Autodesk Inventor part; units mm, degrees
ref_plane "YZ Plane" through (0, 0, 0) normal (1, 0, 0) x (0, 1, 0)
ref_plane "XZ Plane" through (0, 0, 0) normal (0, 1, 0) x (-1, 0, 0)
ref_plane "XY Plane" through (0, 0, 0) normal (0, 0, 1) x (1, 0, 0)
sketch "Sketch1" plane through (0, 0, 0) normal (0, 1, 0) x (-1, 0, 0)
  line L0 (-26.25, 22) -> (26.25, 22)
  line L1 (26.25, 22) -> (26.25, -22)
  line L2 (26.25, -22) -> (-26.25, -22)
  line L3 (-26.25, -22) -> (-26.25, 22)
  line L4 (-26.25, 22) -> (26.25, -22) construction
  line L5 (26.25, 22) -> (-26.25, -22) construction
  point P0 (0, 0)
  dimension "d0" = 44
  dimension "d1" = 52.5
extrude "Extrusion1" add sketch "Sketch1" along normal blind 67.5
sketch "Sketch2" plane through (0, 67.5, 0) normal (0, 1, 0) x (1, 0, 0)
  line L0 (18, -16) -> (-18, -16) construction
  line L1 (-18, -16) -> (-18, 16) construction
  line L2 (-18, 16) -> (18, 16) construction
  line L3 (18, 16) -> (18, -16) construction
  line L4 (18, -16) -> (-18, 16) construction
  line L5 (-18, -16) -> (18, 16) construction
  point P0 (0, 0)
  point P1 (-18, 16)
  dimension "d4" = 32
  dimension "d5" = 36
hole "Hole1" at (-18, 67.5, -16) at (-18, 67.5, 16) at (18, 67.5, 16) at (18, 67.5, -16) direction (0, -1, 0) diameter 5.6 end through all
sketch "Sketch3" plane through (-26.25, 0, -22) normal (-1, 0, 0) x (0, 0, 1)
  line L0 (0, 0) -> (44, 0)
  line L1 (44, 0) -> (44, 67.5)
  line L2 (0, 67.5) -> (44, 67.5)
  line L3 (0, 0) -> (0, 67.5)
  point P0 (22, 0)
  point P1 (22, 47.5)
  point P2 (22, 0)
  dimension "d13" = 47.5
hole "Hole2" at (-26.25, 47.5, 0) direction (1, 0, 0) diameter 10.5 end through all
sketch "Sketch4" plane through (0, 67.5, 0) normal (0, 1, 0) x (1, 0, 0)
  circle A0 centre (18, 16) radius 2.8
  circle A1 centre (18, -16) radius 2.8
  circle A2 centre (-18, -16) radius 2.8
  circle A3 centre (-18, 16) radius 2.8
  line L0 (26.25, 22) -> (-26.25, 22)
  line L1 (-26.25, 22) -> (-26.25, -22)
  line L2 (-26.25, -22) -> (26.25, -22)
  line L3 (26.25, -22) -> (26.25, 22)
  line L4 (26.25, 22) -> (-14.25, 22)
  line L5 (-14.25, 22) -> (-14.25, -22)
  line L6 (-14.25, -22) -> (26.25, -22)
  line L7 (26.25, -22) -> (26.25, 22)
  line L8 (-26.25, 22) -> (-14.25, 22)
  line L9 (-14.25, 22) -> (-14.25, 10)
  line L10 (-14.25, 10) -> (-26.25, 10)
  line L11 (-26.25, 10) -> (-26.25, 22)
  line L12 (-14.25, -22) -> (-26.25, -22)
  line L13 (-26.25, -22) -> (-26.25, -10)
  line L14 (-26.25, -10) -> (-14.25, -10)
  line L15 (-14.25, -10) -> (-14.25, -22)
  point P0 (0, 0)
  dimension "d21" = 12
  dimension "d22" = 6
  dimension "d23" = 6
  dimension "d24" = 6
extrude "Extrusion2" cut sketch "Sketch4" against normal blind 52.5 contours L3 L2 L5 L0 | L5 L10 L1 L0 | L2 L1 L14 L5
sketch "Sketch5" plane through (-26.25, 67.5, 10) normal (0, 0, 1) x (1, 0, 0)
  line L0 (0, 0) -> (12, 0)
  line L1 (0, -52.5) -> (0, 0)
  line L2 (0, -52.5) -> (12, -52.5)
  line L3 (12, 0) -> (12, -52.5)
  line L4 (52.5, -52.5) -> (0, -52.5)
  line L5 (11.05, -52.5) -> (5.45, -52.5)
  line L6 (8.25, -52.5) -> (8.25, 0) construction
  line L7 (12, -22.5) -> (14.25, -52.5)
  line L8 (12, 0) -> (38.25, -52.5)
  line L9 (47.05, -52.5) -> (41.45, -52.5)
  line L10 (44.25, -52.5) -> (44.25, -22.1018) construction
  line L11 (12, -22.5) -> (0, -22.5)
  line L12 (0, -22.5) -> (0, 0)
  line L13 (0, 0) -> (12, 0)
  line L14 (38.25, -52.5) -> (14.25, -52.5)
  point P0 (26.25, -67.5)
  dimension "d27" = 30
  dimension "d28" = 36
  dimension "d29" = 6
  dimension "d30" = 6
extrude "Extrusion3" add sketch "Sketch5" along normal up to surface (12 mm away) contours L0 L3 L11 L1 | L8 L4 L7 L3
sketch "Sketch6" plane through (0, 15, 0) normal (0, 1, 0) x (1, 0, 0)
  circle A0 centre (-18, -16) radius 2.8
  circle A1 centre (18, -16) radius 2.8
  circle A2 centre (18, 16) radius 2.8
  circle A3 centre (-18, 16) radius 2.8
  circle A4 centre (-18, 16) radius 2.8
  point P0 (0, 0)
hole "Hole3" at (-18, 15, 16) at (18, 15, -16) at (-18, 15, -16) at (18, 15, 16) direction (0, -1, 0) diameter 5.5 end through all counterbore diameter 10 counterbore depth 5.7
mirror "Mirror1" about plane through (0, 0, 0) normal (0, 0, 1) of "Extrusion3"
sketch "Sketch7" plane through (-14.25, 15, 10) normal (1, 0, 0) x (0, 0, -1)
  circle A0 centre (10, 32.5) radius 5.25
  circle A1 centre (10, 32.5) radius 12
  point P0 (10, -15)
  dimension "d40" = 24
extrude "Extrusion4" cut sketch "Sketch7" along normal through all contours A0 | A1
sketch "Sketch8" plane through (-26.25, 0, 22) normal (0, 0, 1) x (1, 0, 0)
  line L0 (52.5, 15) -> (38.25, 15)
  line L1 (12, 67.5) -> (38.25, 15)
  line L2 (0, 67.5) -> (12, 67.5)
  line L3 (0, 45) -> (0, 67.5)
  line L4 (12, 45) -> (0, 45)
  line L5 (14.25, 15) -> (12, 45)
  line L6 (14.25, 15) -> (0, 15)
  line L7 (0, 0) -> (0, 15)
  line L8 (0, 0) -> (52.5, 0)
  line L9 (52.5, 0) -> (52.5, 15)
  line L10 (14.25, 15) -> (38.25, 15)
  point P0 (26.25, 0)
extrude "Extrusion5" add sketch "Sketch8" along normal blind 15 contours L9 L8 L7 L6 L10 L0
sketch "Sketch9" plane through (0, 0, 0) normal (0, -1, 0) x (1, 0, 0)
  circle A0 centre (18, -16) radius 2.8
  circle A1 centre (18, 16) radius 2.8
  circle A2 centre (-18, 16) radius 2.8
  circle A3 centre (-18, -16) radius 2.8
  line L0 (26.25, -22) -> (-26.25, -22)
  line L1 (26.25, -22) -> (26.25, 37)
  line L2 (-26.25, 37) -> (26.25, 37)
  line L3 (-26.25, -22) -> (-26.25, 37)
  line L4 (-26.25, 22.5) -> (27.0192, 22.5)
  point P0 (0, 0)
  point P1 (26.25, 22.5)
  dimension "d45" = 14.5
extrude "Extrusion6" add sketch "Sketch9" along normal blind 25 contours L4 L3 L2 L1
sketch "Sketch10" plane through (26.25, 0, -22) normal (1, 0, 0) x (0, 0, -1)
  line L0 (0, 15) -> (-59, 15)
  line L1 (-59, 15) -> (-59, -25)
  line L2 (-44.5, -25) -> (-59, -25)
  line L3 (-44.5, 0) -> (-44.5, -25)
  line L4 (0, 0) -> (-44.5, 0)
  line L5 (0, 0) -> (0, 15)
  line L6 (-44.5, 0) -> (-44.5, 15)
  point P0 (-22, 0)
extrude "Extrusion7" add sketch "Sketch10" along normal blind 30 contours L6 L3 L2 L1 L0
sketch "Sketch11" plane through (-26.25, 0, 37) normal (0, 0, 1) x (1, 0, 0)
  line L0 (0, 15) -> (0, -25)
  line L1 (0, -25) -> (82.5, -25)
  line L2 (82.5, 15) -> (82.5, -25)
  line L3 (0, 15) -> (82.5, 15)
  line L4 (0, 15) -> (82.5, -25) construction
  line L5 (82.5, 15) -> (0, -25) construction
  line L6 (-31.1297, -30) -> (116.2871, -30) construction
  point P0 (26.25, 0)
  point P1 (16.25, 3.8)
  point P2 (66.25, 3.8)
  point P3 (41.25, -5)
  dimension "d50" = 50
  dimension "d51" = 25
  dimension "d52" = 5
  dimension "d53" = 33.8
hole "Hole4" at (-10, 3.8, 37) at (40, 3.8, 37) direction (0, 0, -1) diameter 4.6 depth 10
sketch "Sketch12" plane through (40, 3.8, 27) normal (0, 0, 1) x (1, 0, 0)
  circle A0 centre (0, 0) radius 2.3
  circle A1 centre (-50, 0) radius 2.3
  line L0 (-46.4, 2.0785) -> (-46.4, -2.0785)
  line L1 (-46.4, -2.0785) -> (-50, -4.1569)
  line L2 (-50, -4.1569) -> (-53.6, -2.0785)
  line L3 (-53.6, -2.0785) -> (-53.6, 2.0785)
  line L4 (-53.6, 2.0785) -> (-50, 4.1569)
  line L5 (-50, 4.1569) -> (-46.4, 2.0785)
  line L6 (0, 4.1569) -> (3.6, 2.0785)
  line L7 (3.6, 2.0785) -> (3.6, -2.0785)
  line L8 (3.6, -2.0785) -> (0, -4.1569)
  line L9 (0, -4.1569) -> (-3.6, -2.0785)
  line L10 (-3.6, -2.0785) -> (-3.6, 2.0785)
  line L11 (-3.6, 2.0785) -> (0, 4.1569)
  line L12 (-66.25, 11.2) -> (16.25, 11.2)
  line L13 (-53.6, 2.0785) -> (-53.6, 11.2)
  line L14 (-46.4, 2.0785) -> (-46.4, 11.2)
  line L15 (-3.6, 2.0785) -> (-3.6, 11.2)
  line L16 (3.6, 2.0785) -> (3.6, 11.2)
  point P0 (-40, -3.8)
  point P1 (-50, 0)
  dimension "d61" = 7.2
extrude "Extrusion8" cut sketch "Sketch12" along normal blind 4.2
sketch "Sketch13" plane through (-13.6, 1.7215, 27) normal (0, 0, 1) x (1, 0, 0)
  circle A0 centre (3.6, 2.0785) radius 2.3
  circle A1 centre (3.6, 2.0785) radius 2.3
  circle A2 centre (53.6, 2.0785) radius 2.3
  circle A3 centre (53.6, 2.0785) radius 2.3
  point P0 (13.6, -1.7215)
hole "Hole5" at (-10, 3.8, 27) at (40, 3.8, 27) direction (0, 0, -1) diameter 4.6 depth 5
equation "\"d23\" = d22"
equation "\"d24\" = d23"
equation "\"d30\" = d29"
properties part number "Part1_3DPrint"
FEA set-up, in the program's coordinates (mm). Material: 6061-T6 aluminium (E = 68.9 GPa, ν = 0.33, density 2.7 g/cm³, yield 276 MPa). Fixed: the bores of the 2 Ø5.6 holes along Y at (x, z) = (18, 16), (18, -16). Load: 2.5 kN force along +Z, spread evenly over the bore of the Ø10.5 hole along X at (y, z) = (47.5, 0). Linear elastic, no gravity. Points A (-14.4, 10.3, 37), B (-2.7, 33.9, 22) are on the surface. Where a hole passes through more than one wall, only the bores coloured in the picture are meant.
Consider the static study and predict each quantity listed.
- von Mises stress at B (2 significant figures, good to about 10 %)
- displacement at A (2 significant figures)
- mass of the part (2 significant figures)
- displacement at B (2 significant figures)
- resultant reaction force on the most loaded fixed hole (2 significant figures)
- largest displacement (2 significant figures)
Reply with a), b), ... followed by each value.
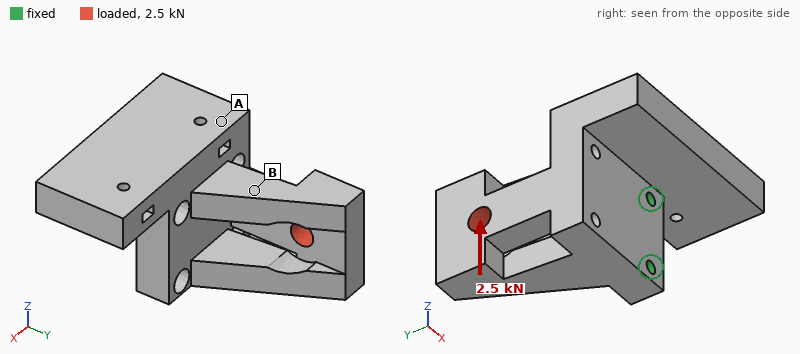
a) 21 MPa
b) 0.033 mm
c) 300 g
d) 0.049 mm
e) 4.2 kN
f) 0.11 mm
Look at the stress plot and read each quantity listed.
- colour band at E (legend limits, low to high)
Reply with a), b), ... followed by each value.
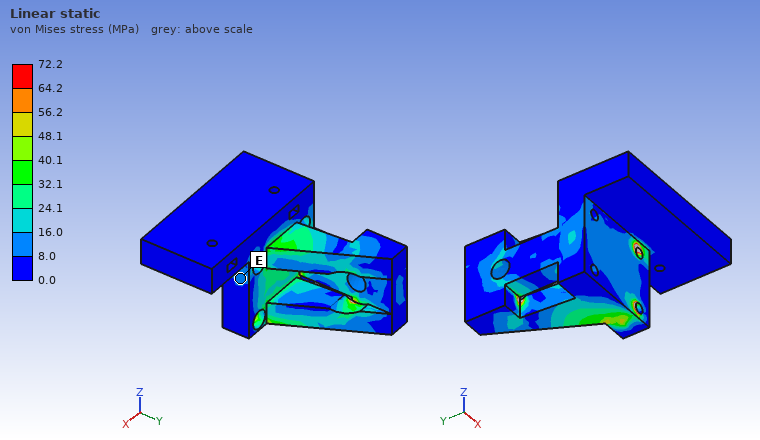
a) 8.0 to 16.0 MPa
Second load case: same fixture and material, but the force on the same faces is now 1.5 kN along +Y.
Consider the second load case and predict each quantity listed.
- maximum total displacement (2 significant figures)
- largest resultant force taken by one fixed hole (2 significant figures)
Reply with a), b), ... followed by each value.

a) 0.13 mm
b) 770 N
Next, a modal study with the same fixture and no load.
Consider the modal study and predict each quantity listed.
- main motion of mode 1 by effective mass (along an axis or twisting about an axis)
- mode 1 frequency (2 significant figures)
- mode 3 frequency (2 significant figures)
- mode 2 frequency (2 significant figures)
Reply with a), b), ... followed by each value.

a) along Y
b) 1600 Hz
c) 4300 Hz
d) 3000 Hz
